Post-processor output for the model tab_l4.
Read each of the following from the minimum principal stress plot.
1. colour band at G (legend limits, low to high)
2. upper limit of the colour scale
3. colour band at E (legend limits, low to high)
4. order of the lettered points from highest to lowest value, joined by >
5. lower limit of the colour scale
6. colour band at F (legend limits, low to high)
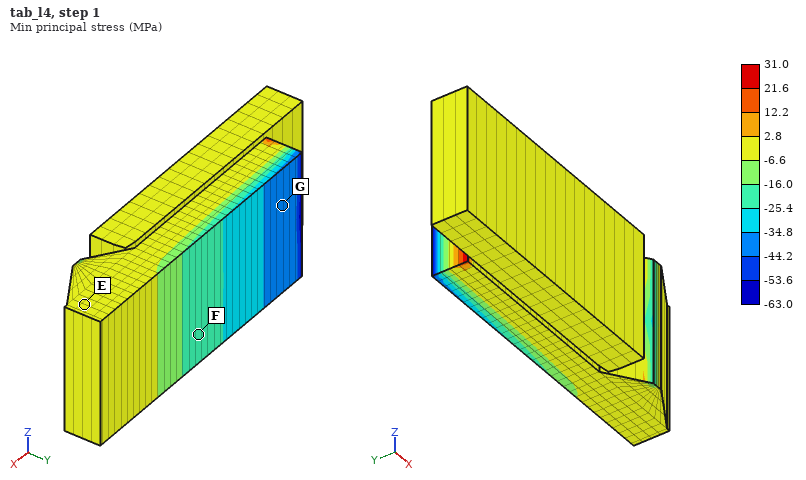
-44.2 to -34.8 MPa
31.0 MPa
-6.6 to 2.8 MPa
E > F > G
-63.0 MPa
-25.4 to -16.0 MPa
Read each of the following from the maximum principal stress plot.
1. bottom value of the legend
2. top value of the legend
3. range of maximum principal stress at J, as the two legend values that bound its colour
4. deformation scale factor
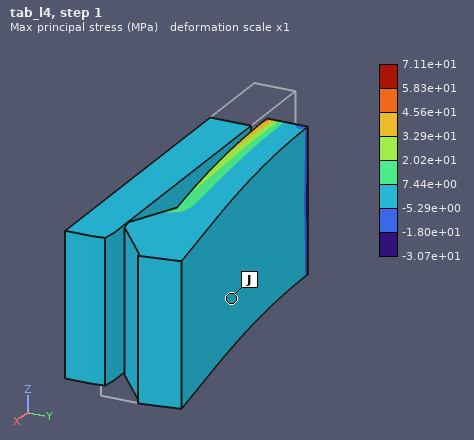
-3.07e+01 MPa
7.11e+01 MPa
-5.29e+00 to 7.44e+00 MPa
1
